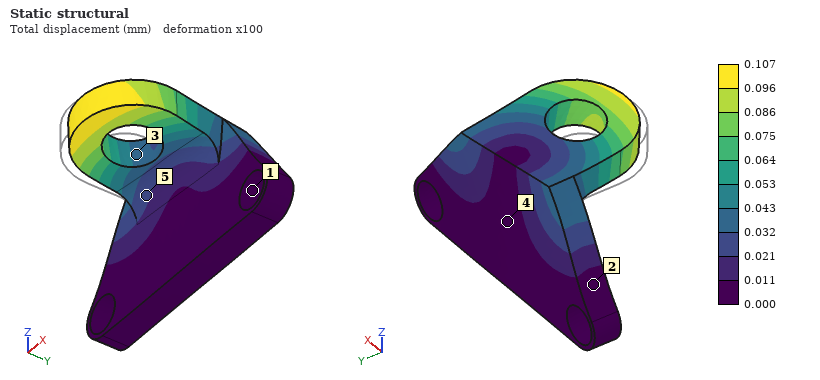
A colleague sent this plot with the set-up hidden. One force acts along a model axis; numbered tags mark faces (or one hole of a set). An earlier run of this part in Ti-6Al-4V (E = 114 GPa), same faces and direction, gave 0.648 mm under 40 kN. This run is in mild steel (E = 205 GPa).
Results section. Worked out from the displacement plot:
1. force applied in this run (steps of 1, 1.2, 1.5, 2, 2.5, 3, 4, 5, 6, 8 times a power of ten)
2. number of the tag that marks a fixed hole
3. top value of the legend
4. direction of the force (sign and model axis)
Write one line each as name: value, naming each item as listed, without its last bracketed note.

force applied in this run: 12 kN
number of the tag that marks a fixed hole: 1
top value of the legend: 0.107 mm
direction of the force: +X
